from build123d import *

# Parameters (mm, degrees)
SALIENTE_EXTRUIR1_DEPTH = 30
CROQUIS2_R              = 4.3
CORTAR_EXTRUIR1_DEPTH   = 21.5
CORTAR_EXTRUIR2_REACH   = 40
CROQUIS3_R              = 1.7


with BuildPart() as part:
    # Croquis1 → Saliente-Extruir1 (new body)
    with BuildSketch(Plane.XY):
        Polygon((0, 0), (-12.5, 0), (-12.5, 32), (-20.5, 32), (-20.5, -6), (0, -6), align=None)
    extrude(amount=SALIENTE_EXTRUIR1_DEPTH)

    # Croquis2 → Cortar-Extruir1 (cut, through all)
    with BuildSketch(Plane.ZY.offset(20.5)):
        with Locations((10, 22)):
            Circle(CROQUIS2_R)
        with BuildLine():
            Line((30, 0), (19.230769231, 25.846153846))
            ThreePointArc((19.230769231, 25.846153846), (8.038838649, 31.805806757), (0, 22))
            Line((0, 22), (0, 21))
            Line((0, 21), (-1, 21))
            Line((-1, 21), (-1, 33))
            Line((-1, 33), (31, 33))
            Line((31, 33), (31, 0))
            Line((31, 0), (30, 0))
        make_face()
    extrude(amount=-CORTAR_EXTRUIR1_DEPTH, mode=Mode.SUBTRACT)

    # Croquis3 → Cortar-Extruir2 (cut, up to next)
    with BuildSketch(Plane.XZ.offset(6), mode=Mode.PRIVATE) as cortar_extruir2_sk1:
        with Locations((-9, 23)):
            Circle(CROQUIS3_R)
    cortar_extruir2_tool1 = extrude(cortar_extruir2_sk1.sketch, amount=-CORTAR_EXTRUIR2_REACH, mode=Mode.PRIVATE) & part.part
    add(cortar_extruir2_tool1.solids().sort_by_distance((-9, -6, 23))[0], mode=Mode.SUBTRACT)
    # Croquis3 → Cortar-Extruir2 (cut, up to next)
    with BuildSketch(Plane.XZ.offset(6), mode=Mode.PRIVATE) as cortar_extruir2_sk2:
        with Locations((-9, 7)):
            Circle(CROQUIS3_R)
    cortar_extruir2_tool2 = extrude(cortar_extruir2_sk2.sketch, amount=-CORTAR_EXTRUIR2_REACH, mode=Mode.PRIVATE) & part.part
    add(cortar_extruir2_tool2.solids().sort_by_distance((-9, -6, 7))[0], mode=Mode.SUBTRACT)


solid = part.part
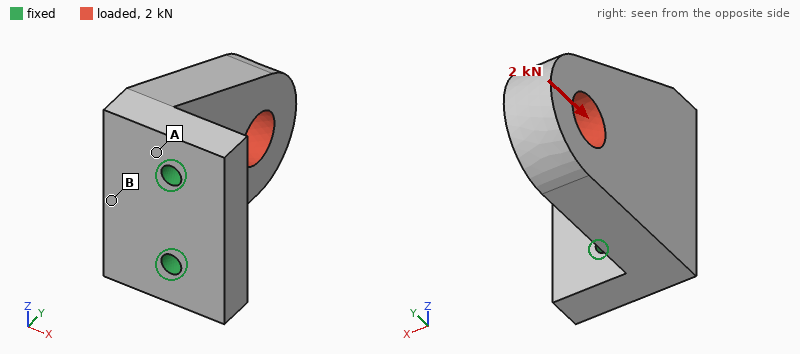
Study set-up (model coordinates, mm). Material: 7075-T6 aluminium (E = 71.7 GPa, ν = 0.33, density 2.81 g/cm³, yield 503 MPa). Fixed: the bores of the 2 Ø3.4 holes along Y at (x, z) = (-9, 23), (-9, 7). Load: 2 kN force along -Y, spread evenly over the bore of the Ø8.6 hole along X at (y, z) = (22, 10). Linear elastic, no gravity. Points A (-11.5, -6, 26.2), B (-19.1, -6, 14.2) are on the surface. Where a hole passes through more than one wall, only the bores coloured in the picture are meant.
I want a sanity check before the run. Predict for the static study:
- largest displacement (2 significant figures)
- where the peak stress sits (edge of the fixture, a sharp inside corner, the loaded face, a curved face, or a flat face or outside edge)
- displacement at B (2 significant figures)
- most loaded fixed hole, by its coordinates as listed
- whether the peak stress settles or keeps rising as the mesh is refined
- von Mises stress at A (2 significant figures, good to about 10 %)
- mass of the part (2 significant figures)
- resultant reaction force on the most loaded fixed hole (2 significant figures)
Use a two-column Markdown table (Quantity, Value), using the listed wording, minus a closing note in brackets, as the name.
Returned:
| Quantity | Value |
|---|---|
| largest displacement | 69 µm |
| where the peak stress sits | edge of the fixture |
| displacement at B | 17 µm |
| most loaded fixed hole, by its coordinates as listed | (-9, 7) |
| whether the peak stress settles or keeps rising as the mesh is refined | keeps rising |
| von Mises stress at A | 34 MPa |
| mass of the part | 25 g |
| resultant reaction force on the most loaded fixed hole | 1.5 kN |
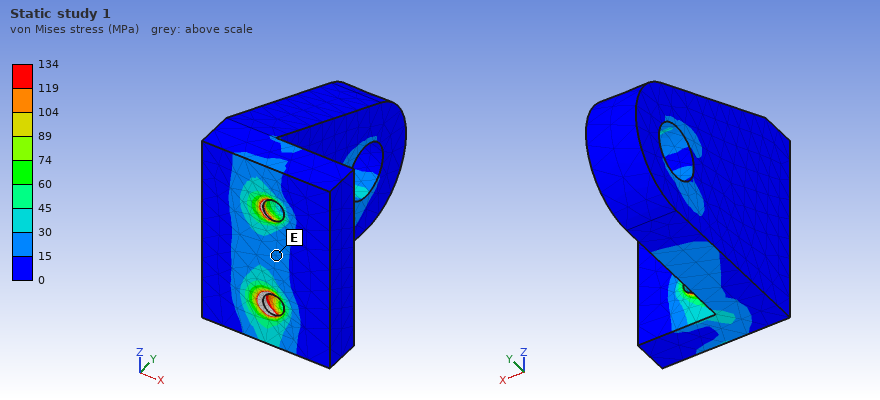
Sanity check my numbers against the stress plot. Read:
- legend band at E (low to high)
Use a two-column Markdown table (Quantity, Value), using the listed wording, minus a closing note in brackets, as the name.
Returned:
| Quantity | Value |
|---|---|
| legend band at E | 15 to 30 MPa |
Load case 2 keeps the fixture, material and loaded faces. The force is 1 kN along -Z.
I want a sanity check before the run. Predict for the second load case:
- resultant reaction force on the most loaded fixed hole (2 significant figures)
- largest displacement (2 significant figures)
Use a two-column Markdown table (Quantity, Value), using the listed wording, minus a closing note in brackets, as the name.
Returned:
| Quantity | Value |
|---|---|
| resultant reaction force on the most loaded fixed hole | 1.4 kN |
| largest displacement | 44 µm |
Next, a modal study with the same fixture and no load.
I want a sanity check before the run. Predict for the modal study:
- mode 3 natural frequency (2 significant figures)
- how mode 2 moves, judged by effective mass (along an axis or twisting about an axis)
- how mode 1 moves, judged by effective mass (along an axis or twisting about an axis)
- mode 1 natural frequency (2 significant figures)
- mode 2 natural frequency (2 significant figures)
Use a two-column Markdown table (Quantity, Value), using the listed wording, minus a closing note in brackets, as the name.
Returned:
| Quantity | Value |
|---|---|
| mode 3 natural frequency | 17 kHz |
| how mode 2 moves, judged by effective mass | along Z |
| how mode 1 moves, judged by effective mass | along X |
| mode 1 natural frequency | 4400 Hz |
| mode 2 natural frequency | 9600 Hz |
